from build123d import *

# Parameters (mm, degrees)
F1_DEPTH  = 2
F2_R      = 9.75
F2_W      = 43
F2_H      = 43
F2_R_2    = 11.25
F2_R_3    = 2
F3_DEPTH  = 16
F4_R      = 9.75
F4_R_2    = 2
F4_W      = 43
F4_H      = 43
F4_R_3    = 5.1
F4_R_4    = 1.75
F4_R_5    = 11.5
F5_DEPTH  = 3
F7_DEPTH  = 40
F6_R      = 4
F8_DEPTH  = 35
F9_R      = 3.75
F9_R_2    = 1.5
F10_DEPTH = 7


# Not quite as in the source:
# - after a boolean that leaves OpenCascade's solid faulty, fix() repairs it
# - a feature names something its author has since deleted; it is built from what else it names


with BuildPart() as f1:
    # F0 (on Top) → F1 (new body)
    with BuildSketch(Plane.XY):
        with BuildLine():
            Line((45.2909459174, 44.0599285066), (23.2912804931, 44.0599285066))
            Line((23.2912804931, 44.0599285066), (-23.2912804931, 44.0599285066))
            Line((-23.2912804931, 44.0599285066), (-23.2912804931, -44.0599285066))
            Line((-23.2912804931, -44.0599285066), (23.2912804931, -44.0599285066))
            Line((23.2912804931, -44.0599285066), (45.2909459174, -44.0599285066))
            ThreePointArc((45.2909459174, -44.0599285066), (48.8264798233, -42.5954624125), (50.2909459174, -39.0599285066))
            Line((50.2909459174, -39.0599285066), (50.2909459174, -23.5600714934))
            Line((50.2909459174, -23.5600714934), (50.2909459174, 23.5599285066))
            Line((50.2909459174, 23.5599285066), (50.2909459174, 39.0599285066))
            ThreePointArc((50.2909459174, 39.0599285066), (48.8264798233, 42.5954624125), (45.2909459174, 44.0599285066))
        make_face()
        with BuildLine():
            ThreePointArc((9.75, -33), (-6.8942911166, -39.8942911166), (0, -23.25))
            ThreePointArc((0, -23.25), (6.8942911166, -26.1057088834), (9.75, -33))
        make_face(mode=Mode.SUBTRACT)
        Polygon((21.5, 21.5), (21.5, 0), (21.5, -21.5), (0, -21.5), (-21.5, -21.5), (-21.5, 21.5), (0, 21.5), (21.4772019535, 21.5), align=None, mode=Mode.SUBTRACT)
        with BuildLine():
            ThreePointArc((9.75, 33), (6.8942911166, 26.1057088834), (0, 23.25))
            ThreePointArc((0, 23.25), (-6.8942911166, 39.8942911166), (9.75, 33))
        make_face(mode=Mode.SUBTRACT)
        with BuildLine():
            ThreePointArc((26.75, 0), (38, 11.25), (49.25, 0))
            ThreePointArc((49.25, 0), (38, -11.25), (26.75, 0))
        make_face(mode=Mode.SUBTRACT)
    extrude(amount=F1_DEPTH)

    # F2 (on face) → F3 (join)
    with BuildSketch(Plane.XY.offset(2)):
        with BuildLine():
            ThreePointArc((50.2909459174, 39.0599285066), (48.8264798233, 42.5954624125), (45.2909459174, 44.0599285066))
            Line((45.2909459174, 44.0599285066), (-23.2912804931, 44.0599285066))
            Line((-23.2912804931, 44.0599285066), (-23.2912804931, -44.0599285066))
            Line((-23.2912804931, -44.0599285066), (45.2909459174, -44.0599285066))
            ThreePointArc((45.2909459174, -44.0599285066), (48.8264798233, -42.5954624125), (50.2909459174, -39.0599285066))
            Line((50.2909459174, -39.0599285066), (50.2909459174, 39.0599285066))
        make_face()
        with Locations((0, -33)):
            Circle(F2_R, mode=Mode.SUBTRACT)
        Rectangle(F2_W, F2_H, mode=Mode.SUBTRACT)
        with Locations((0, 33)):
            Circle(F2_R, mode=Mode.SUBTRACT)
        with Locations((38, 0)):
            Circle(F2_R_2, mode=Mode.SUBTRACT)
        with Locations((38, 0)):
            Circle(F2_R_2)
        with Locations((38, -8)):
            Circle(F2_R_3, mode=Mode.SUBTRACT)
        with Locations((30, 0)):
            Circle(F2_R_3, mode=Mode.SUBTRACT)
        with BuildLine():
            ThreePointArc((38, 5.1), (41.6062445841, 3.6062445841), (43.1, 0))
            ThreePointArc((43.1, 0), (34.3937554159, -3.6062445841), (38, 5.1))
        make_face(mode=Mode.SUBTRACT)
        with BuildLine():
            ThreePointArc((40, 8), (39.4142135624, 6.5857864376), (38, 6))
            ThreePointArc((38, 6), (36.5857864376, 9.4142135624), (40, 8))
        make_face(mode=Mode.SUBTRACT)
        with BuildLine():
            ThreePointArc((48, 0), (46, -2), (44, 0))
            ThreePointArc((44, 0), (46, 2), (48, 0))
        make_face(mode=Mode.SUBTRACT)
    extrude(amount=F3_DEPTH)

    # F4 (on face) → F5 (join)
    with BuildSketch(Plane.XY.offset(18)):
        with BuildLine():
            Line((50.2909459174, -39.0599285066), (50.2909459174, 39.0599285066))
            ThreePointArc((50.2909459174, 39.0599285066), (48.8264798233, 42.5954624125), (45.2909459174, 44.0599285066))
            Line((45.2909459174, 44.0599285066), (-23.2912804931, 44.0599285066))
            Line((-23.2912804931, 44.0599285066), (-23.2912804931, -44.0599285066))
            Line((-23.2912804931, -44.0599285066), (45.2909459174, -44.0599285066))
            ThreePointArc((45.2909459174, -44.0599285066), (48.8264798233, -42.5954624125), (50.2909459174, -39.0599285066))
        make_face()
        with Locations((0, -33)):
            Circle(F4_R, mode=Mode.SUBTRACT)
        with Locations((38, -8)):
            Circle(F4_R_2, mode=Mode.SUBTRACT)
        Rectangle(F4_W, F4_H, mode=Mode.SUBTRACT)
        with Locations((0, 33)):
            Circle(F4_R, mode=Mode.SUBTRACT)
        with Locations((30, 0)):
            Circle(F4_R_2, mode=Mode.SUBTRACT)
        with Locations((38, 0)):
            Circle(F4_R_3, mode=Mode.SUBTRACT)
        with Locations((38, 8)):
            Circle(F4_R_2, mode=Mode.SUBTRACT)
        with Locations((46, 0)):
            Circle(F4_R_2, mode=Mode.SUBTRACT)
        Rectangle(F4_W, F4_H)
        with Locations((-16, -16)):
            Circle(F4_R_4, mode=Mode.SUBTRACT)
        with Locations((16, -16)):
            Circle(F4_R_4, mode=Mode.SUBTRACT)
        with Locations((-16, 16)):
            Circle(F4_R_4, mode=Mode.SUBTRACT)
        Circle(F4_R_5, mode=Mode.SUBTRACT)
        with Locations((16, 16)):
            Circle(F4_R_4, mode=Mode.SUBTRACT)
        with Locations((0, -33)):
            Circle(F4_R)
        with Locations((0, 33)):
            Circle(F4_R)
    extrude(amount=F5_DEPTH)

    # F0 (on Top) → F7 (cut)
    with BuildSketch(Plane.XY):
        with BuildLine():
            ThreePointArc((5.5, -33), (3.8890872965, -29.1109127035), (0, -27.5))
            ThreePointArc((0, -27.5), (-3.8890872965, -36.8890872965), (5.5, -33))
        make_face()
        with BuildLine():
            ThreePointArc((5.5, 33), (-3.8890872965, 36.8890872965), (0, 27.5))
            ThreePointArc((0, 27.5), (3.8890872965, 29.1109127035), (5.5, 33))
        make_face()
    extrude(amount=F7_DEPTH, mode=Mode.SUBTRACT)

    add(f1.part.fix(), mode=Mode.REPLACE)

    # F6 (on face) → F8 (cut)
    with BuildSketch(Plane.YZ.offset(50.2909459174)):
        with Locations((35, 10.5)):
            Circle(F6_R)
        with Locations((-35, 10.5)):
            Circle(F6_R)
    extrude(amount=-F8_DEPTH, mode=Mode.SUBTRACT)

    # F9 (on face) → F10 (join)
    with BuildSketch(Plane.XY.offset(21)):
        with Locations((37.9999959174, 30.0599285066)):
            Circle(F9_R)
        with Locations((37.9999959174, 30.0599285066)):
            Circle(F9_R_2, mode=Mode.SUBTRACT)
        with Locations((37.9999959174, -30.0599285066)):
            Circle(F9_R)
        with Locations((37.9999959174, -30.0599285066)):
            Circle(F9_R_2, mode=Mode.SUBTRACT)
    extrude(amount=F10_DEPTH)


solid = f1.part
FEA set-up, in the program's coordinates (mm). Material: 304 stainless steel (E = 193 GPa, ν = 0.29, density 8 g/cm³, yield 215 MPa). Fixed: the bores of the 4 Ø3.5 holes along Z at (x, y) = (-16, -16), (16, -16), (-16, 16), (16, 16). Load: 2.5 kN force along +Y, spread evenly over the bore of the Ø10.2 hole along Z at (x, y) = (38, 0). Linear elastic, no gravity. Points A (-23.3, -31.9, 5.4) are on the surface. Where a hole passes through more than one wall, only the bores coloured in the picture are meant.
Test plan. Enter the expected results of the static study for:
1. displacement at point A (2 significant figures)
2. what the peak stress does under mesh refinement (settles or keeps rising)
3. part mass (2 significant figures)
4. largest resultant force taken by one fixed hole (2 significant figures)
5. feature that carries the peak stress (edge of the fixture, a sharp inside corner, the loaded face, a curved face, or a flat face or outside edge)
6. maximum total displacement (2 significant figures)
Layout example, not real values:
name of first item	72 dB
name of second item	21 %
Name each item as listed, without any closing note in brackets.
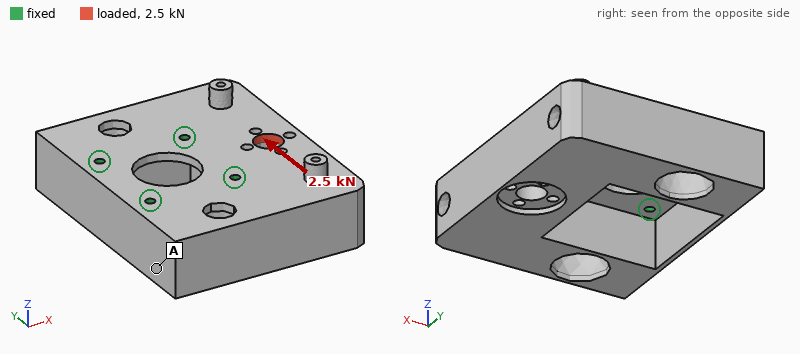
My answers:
displacement at point A	2.3 µm
what the peak stress does under mesh refinement	keeps rising
part mass	670 g
largest resultant force taken by one fixed hole	1.7 kN
feature that carries the peak stress	edge of the fixture
maximum total displacement	6.2 µm
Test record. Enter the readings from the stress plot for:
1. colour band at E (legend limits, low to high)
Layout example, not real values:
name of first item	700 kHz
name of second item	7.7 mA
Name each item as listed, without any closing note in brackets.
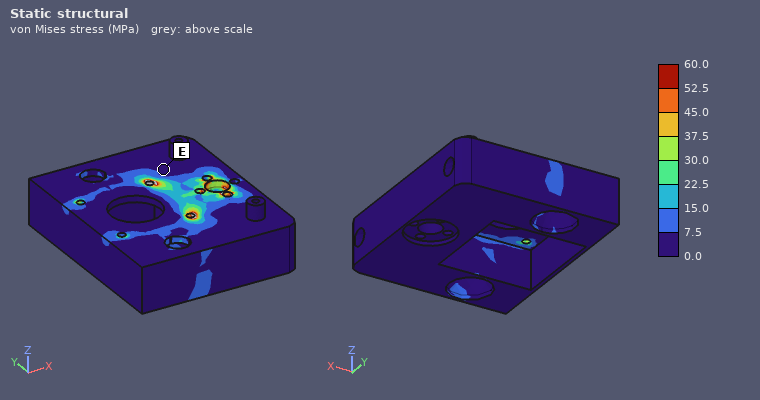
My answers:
colour band at E	0.0 to 7.5 MPa
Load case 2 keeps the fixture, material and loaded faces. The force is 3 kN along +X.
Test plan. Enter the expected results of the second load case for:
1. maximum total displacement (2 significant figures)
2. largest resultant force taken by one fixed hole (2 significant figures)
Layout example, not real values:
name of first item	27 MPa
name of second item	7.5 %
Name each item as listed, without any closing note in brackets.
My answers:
maximum total displacement	6.0 µm
largest resultant force taken by one fixed hole	1.3 kN
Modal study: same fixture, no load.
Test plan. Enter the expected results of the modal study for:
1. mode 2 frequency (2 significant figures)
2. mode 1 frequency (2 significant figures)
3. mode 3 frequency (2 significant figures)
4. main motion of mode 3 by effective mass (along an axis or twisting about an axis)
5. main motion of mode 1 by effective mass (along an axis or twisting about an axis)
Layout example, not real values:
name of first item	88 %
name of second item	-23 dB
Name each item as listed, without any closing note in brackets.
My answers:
mode 2 frequency	2800 Hz
mode 1 frequency	2600 Hz
mode 3 frequency	5200 Hz
main motion of mode 3 by effective mass	along Y
main motion of mode 1 by effective mass	along Z
